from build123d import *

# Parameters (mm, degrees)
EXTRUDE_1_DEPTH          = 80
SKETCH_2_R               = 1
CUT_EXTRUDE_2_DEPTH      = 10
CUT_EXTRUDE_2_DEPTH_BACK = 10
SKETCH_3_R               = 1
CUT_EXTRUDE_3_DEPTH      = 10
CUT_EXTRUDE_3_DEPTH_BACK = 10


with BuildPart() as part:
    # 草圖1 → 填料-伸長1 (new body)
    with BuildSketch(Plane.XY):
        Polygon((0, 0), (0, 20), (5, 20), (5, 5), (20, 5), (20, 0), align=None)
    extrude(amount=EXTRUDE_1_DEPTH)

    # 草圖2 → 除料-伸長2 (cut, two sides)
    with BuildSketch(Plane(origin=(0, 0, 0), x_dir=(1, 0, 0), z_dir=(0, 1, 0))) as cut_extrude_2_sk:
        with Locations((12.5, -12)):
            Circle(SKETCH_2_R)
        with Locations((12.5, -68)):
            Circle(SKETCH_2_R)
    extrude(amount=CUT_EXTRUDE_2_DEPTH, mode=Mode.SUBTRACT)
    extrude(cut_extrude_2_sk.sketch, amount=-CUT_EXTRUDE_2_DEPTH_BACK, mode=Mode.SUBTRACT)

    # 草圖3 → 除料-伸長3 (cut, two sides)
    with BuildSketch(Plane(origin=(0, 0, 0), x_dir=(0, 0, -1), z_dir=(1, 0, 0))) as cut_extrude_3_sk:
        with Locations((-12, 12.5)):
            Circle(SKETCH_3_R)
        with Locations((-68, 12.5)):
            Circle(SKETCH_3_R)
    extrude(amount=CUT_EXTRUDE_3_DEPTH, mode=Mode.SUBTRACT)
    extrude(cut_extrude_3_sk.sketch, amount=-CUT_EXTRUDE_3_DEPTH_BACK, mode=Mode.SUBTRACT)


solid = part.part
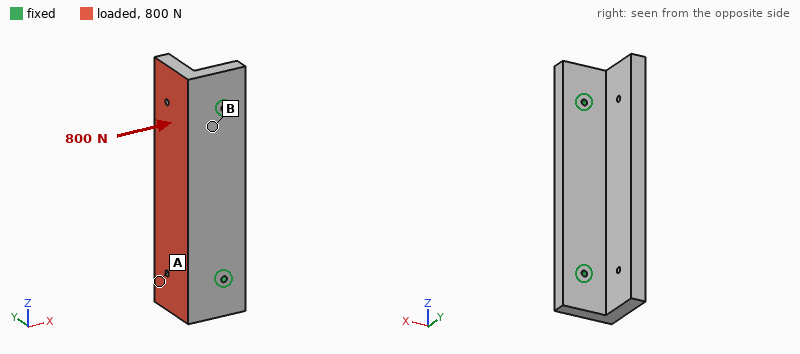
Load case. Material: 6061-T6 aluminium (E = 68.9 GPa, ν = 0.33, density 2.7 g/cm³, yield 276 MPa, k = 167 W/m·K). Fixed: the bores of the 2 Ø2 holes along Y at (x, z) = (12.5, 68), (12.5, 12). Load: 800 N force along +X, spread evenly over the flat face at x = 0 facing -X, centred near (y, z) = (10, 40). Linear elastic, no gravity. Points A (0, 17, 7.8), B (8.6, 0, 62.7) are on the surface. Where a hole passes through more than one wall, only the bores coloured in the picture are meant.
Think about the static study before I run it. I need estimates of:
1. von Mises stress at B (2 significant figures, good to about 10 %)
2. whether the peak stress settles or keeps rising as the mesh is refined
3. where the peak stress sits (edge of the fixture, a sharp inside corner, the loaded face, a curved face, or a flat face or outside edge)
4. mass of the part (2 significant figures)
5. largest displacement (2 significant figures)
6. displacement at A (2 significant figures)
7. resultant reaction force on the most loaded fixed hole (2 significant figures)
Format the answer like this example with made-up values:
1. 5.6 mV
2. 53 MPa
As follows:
1. 17 MPa
2. keeps rising
3. edge of the fixture
4. 38 g
5. 55 µm
6. 40 µm
7. 410 N
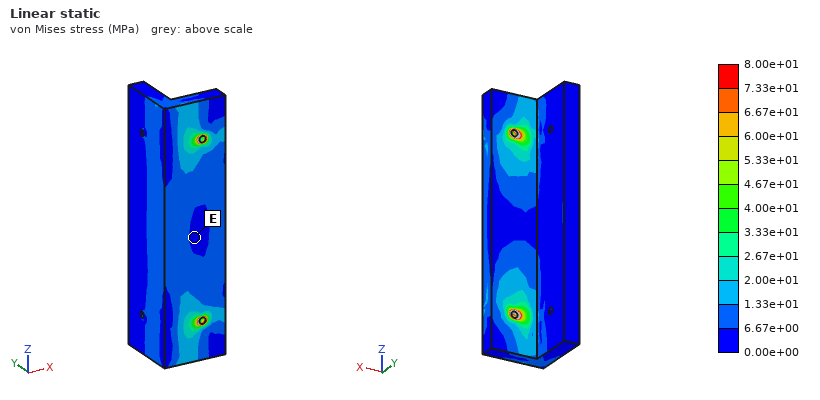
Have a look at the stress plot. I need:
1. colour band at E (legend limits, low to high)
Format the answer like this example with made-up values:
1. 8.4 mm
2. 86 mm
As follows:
1. 0.00e+00 to 6.67e+00 MPa
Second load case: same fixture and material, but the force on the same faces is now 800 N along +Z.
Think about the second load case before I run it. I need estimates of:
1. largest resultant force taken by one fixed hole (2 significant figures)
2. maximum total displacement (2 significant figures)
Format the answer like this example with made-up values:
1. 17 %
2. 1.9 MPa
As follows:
1. 450 N
2. 6.2 µm
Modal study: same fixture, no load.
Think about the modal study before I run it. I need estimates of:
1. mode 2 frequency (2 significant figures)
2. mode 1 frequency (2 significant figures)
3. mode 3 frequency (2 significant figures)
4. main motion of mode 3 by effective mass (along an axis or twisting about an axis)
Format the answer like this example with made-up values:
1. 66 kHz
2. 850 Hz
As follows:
1. 7200 Hz
2. 4400 Hz
3. 9100 Hz
4. along Y
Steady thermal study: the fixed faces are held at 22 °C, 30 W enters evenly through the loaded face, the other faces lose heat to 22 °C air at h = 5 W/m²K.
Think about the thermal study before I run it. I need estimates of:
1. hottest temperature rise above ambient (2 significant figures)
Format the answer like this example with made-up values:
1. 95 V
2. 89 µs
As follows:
1. 15 K
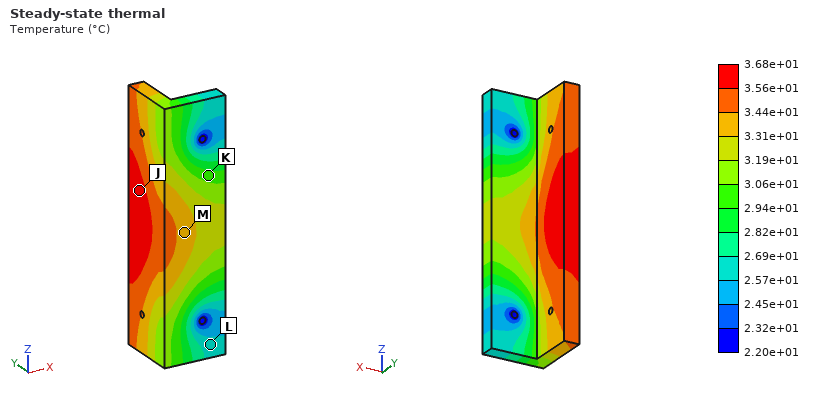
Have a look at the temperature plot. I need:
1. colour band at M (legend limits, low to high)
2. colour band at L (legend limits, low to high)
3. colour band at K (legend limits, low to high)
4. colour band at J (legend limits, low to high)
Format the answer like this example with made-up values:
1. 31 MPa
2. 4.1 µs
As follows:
1. 3.31e+01 to 3.44e+01 °C
2. 2.57e+01 to 2.69e+01 °C
3. 2.94e+01 to 3.06e+01 °C
4. 3.56e+01 to 3.68e+01 °C
